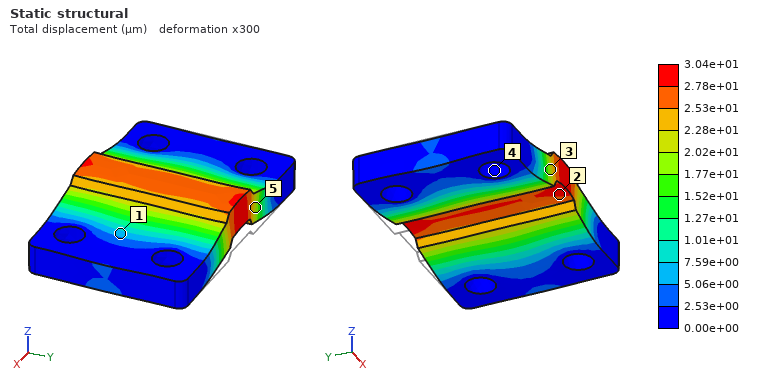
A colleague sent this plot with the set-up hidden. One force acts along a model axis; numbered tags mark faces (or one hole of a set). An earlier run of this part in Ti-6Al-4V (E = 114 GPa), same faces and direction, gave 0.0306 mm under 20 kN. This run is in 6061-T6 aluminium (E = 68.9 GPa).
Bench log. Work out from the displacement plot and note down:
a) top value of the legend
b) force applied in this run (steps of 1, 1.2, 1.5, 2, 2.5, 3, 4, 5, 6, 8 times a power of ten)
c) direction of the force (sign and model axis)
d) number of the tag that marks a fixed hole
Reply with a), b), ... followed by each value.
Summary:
a) 3.04e+01 µm
b) 12 kN
c) +Z
d) 4
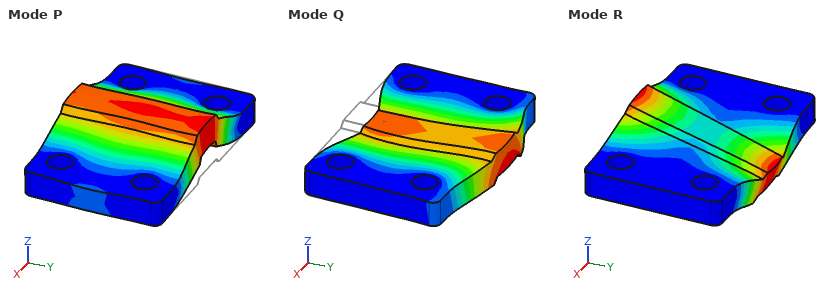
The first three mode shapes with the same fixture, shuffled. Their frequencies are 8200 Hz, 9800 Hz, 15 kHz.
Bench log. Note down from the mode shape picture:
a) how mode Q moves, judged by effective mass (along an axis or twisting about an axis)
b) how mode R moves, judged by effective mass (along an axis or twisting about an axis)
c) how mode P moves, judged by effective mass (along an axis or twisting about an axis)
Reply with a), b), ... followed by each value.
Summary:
a) along Y
b) twisting about X
c) along Z
